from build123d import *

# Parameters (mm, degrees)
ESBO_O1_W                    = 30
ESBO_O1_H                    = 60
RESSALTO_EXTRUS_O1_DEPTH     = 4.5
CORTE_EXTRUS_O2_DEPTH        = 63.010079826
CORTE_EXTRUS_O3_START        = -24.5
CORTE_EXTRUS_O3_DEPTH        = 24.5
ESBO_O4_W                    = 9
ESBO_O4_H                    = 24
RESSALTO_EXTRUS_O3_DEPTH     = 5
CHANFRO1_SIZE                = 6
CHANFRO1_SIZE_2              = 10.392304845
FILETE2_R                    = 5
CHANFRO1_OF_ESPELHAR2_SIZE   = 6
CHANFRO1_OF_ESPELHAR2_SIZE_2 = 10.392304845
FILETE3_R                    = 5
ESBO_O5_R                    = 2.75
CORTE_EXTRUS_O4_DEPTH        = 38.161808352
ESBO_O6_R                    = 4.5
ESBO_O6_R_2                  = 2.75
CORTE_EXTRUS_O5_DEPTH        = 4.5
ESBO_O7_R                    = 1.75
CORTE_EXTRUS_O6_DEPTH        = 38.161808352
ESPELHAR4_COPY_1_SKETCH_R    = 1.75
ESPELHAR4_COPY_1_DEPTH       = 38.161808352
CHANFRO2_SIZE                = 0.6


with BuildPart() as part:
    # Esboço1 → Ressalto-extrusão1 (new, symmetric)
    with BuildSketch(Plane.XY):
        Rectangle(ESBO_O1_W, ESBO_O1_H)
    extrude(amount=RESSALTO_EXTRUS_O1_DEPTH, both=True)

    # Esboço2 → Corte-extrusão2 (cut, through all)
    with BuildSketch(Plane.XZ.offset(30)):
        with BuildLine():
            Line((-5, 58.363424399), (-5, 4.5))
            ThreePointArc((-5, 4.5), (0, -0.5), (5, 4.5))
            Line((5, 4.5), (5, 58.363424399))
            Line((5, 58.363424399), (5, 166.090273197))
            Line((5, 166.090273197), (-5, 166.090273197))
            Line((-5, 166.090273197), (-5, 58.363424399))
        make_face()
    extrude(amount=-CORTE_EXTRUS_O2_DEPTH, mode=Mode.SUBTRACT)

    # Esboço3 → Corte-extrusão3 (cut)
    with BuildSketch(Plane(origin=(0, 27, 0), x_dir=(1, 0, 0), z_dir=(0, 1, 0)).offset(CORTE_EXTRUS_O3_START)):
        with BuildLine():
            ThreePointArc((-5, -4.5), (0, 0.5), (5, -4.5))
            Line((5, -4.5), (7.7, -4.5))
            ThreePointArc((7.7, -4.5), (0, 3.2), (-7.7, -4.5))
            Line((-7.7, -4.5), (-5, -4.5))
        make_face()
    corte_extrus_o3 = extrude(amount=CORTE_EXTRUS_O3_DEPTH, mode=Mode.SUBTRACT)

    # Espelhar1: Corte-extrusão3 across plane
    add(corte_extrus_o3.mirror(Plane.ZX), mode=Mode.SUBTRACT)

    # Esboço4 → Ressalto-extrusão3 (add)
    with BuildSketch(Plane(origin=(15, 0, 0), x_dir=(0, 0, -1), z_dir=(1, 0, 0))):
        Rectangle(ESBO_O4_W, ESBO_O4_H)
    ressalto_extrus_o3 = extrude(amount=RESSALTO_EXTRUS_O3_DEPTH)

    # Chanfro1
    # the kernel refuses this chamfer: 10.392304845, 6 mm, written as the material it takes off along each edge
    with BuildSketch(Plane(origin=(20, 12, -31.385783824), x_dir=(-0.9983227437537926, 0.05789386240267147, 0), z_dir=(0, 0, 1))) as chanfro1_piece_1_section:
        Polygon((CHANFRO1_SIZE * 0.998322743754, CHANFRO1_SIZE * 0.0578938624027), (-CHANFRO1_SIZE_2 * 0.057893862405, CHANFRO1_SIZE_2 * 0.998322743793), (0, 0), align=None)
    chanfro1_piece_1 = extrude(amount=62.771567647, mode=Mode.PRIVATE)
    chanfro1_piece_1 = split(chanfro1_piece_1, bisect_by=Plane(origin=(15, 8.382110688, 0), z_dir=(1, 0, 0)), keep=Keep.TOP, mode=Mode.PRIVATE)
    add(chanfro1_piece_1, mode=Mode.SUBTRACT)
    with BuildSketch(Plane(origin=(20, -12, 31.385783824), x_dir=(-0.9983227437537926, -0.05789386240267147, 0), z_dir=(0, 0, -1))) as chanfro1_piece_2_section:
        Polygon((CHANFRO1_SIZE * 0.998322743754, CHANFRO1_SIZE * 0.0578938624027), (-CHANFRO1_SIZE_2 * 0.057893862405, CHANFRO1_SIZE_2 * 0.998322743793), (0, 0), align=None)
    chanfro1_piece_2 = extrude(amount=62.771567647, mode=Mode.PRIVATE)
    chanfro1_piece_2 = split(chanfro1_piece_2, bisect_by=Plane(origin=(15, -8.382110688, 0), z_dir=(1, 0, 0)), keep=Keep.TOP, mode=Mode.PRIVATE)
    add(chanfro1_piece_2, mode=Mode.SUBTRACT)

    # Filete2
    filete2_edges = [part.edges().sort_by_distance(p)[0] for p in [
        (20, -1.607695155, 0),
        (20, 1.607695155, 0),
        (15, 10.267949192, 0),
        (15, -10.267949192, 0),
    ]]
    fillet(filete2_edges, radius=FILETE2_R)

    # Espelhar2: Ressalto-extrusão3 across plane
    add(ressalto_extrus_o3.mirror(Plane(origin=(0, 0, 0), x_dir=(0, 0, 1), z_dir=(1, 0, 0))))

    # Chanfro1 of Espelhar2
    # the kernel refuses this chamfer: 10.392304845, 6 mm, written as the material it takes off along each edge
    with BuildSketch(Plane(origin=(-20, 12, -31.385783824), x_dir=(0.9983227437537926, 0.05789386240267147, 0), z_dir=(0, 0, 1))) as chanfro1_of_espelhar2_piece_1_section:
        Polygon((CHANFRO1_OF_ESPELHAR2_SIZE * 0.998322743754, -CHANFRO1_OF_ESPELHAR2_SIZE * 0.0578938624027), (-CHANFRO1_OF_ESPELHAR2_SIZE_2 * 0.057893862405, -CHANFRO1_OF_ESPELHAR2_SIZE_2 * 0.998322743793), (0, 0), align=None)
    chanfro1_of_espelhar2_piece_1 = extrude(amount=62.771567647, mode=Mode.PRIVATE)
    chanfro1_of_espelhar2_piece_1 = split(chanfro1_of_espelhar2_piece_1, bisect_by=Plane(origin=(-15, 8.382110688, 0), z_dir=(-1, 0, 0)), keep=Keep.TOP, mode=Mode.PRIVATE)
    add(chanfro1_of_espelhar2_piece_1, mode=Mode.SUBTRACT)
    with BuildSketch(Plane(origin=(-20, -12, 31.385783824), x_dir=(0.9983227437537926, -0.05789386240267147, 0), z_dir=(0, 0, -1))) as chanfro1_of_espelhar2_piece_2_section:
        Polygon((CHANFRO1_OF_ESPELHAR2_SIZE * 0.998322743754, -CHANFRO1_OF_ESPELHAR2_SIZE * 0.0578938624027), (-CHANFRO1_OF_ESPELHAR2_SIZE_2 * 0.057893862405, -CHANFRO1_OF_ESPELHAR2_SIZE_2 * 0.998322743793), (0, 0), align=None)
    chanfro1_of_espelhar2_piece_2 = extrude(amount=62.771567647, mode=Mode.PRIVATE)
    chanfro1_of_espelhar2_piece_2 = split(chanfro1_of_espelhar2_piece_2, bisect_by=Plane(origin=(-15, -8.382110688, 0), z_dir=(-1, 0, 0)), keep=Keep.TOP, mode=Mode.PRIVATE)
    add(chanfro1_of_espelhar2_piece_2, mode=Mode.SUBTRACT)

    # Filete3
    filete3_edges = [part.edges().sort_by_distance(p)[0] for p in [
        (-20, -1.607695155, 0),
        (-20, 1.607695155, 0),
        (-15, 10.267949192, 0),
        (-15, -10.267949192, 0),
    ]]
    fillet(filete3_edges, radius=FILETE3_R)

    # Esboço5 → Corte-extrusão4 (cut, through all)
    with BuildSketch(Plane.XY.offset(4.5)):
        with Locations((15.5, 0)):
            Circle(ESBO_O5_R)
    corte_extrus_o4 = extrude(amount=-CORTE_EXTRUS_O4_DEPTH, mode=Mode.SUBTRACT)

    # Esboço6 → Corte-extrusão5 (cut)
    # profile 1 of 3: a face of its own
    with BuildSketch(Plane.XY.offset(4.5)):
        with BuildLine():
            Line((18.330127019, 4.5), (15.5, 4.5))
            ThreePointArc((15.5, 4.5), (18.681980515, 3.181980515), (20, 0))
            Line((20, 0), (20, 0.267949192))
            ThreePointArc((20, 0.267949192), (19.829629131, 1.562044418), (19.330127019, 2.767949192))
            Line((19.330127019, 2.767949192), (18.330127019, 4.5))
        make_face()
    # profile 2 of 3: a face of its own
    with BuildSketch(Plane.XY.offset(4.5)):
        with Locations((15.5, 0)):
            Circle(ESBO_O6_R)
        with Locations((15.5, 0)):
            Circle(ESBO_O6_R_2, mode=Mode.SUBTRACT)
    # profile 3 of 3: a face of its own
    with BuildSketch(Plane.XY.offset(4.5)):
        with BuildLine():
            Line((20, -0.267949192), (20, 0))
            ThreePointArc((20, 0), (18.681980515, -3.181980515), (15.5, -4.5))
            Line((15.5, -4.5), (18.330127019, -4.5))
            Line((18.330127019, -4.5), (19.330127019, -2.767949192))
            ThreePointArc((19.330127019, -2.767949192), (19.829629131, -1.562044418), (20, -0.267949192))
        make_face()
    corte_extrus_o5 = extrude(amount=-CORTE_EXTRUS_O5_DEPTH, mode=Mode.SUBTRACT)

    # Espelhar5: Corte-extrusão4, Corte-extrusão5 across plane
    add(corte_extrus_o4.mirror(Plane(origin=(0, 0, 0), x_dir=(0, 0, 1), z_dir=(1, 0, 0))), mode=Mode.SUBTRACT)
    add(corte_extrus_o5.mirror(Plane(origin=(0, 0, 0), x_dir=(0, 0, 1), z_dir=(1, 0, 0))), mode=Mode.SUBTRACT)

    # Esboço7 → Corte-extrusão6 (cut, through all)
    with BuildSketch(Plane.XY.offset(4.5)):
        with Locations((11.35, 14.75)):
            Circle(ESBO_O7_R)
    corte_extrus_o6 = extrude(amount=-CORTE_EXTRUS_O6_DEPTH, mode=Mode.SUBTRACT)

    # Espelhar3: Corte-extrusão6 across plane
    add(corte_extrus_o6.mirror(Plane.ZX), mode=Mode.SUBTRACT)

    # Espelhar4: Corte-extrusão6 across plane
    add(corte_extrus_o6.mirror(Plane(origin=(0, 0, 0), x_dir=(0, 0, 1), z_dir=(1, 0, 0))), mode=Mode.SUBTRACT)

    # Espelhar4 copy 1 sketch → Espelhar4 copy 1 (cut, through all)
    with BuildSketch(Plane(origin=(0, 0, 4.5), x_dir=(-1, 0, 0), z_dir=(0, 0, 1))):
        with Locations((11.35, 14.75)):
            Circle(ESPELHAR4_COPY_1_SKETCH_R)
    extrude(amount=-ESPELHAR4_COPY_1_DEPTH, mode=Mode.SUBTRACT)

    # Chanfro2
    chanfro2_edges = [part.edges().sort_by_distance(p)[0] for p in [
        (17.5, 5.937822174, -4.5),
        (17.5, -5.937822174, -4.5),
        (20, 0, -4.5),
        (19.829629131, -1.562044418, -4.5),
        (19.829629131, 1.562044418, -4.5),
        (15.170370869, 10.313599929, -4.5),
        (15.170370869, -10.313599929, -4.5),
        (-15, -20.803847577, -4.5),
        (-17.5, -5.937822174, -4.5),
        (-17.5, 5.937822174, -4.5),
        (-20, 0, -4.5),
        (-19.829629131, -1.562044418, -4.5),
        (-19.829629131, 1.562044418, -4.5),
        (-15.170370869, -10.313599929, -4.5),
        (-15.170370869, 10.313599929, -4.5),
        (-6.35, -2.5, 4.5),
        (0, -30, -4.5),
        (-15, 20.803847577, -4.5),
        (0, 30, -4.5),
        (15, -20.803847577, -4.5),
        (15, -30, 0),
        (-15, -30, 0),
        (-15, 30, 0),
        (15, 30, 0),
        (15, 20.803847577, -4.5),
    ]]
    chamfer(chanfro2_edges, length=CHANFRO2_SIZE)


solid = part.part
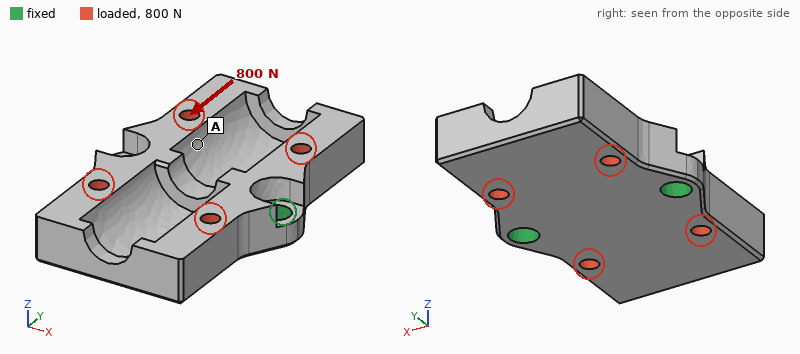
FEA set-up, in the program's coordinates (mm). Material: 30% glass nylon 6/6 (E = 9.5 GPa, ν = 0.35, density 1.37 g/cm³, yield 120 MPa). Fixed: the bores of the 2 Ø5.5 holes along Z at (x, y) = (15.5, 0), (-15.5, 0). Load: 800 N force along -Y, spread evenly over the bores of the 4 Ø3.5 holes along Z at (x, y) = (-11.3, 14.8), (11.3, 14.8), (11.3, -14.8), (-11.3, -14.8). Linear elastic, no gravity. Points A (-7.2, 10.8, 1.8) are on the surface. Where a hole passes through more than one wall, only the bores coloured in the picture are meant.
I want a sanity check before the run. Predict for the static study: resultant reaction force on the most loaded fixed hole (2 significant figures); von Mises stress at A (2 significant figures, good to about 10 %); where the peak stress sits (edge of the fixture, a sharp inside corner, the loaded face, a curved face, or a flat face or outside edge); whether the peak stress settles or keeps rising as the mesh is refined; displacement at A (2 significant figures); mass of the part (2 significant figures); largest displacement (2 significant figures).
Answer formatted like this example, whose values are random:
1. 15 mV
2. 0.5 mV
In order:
1. 400 N
2. 2.3 MPa
3. edge of the fixture
4. keeps rising
5. 21 µm
6. 15 g
7. 55 µm
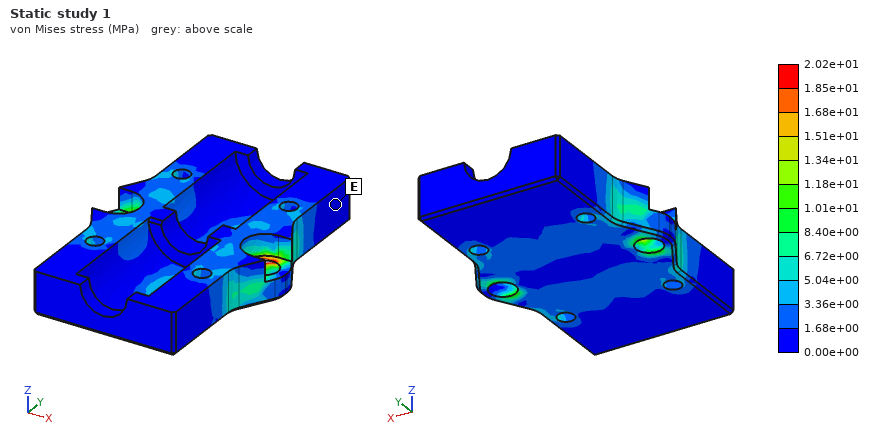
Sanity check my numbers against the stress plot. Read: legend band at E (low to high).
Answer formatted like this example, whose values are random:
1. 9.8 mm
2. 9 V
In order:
1. 0.00e+00 to 1.68e+00 MPa
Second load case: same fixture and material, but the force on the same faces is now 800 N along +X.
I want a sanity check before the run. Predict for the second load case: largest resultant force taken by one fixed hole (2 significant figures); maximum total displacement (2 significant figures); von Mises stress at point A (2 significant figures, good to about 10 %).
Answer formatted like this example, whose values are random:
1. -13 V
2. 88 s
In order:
1. 400 N
2. 31 µm
3. 2.9 MPa
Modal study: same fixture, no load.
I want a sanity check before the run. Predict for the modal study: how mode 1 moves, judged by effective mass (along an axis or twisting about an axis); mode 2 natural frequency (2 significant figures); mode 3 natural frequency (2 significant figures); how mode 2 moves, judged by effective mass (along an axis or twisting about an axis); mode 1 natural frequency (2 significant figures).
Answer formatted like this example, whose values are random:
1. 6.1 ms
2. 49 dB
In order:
1. twisting about X
2. 3500 Hz
3. 5000 Hz
4. along Z
5. 2200 Hz
